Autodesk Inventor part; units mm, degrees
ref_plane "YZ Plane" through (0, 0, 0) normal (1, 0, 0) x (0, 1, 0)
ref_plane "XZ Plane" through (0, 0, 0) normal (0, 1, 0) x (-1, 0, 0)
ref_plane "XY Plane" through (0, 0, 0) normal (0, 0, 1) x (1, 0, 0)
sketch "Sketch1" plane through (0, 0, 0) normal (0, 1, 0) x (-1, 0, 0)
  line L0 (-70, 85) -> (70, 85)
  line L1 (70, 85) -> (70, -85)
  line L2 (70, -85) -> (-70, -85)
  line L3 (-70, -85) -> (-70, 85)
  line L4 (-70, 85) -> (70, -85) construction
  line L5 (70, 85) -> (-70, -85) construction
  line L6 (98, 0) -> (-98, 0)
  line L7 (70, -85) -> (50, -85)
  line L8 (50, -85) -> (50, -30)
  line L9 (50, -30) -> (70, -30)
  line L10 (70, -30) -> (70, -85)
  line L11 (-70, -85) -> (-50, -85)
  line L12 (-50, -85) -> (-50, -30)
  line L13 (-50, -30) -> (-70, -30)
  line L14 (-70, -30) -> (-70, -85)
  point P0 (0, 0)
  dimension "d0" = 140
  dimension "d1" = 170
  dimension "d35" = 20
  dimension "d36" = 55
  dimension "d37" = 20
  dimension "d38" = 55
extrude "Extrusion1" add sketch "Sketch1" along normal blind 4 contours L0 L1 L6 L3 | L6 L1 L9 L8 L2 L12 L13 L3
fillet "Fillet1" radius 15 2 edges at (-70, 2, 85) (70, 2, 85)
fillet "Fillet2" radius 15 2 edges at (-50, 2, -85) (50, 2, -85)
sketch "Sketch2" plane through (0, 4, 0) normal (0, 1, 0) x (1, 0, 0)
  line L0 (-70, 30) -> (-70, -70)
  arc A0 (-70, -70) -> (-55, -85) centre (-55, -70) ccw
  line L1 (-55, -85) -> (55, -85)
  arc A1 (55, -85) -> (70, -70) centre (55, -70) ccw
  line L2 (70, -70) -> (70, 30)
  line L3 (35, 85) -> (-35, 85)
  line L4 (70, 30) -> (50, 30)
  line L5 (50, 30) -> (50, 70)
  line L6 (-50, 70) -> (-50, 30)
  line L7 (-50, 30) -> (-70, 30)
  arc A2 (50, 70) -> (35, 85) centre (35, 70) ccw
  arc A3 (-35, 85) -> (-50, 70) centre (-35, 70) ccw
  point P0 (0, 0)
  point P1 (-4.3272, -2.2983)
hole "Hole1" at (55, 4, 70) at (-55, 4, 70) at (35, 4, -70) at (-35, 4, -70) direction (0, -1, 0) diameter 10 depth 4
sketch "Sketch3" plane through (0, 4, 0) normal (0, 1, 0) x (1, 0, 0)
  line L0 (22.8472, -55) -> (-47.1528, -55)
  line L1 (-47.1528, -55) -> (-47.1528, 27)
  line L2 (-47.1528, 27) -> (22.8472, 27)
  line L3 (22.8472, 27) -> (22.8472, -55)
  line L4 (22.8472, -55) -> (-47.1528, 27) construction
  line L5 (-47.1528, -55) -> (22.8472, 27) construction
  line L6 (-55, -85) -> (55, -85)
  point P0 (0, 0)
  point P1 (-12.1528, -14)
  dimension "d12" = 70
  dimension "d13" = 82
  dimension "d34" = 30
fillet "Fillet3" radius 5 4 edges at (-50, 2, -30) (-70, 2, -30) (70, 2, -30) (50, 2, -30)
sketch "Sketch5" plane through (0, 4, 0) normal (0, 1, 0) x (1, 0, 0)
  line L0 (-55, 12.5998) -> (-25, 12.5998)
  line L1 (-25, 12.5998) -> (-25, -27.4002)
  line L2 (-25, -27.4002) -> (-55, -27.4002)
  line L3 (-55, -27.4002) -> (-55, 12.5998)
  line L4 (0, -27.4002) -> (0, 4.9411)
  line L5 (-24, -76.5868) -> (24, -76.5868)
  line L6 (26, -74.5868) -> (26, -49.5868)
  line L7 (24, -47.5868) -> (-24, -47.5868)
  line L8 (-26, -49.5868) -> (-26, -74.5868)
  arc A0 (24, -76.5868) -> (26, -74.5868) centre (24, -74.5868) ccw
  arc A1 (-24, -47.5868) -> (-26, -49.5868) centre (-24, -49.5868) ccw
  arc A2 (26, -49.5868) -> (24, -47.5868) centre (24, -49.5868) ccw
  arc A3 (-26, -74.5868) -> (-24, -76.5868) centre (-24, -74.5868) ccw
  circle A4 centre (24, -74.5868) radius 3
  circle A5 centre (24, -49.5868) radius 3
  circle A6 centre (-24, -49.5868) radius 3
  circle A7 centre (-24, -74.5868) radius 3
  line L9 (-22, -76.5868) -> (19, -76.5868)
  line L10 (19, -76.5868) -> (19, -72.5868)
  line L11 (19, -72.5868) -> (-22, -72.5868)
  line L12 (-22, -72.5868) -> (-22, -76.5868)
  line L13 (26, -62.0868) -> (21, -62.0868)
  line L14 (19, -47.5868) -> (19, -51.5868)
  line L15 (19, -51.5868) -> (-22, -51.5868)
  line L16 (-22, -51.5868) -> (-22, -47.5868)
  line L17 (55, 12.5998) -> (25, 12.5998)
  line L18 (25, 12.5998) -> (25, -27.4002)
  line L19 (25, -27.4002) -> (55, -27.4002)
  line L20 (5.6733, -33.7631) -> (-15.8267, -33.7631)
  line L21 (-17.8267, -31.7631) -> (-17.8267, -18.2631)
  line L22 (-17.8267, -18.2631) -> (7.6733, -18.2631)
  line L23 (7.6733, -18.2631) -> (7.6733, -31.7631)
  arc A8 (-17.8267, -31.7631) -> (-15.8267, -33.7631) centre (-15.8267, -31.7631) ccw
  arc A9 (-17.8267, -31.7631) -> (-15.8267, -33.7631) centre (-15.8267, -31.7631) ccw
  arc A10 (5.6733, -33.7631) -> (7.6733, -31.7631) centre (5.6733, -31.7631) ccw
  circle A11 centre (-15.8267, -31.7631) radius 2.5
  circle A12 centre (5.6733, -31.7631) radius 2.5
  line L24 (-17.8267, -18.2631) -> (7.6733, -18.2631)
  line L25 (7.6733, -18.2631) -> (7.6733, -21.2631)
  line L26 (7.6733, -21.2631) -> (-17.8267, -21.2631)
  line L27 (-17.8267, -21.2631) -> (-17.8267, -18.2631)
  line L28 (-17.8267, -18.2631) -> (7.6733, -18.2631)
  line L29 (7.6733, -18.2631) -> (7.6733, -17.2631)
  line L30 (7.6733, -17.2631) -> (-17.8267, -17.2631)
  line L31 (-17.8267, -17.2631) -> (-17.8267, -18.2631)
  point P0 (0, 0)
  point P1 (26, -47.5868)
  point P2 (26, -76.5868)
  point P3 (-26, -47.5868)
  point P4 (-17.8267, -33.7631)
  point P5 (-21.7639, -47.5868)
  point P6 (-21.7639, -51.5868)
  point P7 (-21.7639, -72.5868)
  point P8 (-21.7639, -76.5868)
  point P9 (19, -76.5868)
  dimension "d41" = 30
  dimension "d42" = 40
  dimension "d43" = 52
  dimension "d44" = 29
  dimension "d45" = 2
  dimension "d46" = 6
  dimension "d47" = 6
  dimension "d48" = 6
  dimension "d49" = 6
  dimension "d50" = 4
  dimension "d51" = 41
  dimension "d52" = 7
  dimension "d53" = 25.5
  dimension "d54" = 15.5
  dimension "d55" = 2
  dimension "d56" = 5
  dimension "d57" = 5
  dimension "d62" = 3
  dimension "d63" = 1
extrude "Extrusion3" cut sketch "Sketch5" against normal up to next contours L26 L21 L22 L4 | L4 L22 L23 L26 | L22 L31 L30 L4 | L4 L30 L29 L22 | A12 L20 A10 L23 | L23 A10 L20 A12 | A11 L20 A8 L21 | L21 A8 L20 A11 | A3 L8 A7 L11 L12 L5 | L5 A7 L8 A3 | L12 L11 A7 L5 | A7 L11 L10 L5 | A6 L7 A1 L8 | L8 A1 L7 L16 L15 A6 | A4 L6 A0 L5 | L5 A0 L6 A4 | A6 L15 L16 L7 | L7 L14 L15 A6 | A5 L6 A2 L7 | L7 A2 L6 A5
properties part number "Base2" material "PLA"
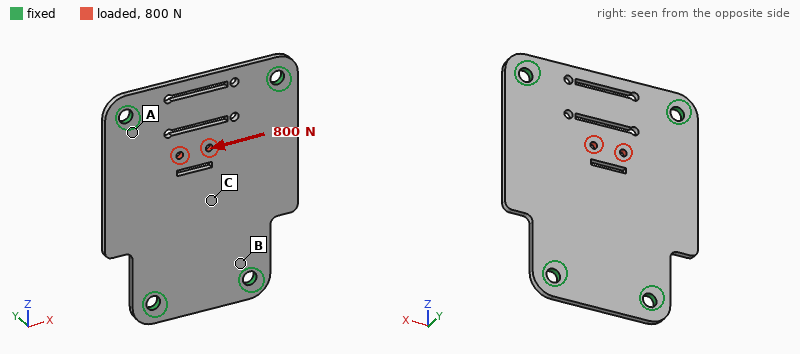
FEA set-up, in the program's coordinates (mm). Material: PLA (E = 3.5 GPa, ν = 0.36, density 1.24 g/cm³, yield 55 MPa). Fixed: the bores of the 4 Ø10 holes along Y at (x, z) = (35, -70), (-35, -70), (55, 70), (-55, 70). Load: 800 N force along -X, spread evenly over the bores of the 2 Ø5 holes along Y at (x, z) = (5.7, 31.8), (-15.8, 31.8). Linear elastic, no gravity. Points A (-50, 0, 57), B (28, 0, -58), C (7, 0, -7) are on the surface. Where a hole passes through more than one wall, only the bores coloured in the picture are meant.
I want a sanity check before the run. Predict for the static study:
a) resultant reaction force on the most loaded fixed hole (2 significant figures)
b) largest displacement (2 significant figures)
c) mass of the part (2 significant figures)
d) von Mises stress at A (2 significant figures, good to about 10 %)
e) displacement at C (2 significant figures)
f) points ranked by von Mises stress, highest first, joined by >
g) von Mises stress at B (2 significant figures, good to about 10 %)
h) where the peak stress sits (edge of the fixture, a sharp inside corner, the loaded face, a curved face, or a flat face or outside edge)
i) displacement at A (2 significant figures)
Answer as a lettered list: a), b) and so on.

a) 290 N
b) 88 µm
c) 100 g
d) 3.2 MPa
e) 42 µm
f) A > B > C
g) 1.8 MPa
h) a curved face
i) 22 µm
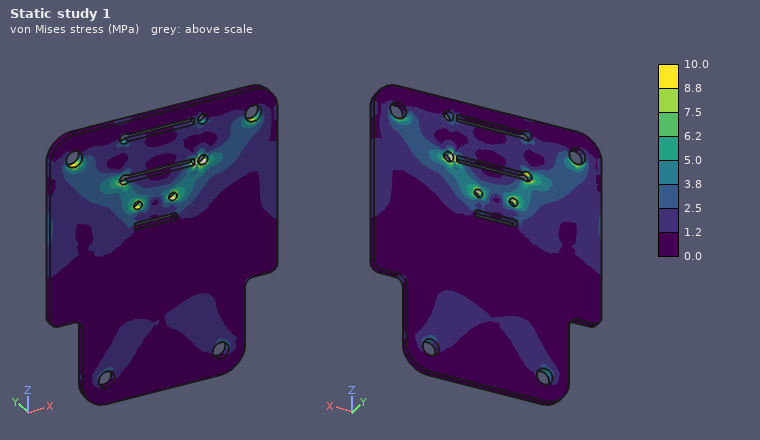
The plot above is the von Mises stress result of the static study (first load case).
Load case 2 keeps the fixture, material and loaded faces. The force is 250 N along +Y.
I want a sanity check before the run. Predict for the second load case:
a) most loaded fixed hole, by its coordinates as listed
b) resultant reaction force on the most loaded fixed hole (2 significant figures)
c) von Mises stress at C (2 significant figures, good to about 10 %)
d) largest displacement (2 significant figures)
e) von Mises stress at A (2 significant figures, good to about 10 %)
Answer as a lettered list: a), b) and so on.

a) (-55, 70)
b) 110 N
c) 5.7 MPa
d) 2.4 mm
e) 15 MPa
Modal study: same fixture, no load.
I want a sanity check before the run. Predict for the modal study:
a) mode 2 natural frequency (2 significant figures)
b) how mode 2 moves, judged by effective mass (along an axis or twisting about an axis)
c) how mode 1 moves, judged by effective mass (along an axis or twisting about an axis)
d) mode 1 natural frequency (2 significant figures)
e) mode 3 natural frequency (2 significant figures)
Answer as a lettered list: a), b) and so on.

a) 390 Hz
b) twisting about Z
c) along Y
d) 320 Hz
e) 540 Hz
